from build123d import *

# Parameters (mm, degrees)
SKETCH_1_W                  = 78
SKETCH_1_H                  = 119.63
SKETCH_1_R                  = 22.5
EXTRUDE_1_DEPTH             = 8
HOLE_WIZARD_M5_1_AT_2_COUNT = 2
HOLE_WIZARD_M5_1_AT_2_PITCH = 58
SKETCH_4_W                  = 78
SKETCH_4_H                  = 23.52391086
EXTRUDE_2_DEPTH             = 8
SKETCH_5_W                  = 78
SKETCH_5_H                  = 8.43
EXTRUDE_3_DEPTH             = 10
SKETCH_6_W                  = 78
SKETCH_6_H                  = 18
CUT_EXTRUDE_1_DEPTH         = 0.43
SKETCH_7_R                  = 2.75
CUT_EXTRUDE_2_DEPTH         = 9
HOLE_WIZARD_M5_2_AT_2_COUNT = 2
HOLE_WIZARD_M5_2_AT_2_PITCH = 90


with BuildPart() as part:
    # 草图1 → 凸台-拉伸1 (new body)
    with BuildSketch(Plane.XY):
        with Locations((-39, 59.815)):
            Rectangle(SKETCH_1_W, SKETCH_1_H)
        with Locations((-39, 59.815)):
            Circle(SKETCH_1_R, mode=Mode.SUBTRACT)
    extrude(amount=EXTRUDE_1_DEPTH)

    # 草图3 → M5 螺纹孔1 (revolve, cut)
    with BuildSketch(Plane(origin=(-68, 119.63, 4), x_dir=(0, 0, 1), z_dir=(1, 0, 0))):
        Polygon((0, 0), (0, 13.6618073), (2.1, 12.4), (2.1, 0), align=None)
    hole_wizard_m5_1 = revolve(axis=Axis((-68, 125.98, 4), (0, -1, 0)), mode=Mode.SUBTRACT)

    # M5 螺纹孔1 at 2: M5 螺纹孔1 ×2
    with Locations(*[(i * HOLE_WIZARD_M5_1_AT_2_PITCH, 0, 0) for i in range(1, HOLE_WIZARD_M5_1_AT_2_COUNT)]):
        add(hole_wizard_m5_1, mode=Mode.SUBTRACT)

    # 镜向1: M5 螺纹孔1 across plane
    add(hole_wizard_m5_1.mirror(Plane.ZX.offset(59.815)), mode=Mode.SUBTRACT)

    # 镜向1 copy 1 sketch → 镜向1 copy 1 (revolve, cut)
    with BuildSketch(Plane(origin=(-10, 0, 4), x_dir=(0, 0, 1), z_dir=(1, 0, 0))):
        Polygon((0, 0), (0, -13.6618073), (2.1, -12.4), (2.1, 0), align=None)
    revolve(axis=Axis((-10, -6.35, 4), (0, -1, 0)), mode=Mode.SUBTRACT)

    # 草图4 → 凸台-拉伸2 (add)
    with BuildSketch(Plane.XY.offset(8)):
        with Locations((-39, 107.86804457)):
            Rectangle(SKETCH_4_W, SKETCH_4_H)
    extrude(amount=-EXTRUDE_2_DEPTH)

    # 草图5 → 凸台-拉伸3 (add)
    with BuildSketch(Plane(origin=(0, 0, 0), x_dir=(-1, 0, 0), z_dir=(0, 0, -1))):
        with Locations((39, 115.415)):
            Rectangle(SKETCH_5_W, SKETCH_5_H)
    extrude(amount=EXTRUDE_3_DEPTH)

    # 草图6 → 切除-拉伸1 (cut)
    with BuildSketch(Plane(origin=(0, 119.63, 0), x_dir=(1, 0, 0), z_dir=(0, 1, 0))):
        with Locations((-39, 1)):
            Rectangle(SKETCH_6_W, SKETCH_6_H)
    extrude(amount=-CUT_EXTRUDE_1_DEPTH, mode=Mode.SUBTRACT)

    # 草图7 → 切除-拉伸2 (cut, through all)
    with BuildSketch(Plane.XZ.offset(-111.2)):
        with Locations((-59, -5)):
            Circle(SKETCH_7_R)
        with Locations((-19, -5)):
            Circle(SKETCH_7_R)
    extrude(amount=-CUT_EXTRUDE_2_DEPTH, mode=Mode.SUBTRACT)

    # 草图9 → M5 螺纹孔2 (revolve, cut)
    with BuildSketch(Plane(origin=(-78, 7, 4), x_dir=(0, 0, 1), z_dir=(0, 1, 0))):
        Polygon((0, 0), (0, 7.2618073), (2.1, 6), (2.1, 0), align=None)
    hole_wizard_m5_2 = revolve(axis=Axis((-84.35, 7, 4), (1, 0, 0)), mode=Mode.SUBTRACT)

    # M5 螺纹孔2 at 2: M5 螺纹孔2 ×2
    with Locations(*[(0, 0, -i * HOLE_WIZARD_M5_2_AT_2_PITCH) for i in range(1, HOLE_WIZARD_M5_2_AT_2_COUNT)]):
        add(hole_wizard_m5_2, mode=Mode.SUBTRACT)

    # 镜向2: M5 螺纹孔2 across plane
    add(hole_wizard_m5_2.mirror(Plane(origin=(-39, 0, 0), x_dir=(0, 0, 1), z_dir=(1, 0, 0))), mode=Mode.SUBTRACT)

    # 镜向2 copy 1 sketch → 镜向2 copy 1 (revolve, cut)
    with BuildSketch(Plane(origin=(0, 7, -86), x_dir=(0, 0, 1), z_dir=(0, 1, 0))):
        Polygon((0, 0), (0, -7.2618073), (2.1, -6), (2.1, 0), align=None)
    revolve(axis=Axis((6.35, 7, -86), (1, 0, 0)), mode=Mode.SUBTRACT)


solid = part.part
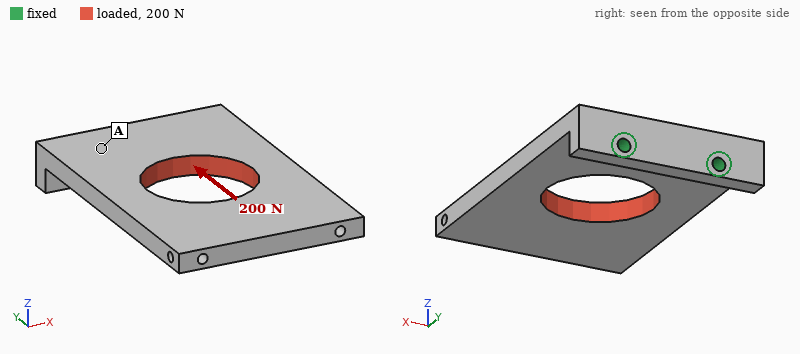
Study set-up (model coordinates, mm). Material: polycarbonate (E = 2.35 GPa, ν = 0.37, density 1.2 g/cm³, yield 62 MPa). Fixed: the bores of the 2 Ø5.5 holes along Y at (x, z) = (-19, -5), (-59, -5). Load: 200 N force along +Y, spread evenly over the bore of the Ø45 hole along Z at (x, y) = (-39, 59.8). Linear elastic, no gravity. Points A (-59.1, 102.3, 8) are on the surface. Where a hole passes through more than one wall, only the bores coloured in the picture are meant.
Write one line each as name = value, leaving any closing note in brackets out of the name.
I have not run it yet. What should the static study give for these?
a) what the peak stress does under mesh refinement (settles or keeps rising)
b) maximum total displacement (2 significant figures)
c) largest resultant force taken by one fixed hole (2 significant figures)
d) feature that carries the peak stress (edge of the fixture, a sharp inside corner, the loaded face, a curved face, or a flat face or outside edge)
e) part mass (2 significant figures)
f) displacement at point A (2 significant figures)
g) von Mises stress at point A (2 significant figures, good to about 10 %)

what the peak stress does under mesh refinement = keeps rising
maximum total displacement = 0.23 mm
largest resultant force taken by one fixed hole = 100 N
feature that carries the peak stress = edge of the fixture
part mass = 80 g
displacement at point A = 0.037 mm
von Mises stress at point A = 0.48 MPa
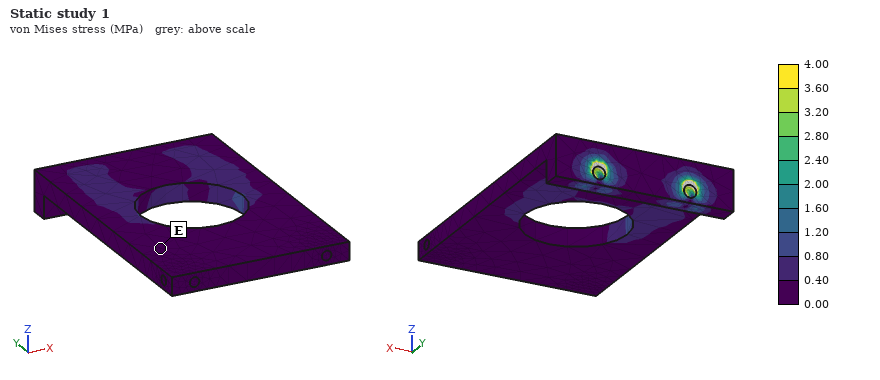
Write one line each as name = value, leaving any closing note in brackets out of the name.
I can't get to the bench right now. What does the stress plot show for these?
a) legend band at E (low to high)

legend band at E = 0.00 to 0.40 MPa
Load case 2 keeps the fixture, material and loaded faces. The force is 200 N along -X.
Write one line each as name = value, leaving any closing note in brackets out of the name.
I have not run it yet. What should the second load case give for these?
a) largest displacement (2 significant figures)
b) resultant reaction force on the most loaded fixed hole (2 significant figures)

largest displacement = 0.35 mm
resultant reaction force on the most loaded fixed hole = 270 N
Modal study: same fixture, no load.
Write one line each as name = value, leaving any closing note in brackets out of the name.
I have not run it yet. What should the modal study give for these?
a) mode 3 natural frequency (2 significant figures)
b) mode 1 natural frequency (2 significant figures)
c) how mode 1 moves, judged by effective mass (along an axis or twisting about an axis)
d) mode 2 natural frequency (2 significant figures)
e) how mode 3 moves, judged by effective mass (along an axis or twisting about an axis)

mode 3 natural frequency = 530 Hz
mode 1 natural frequency = 110 Hz
how mode 1 moves, judged by effective mass = along Z
mode 2 natural frequency = 360 Hz
how mode 3 moves, judged by effective mass = along X
